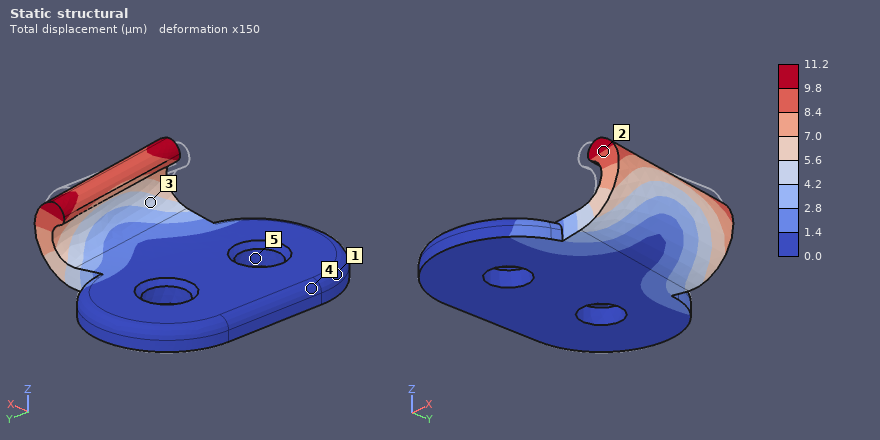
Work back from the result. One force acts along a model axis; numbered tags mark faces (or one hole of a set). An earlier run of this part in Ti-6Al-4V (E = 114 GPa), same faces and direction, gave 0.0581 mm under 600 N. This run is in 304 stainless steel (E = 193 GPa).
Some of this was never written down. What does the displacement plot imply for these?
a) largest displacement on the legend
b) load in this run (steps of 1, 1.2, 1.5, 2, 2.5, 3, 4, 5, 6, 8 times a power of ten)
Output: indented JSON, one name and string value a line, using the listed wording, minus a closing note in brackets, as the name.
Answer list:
{
  "largest displacement on the legend": "11.2 µm",
  "load in this run": "200 N"
}
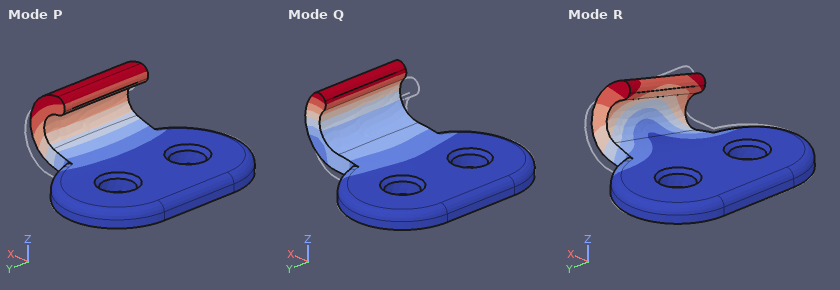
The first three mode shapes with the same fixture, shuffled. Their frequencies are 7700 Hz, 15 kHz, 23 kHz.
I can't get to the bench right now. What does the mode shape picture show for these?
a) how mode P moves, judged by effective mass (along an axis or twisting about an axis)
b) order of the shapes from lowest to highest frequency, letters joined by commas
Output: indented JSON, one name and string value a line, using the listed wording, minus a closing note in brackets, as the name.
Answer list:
{
  "how mode P moves, judged by effective mass": "along Z",
  "order of the shapes from lowest to highest frequency, letters joined by commas": "P, R, Q"
}
